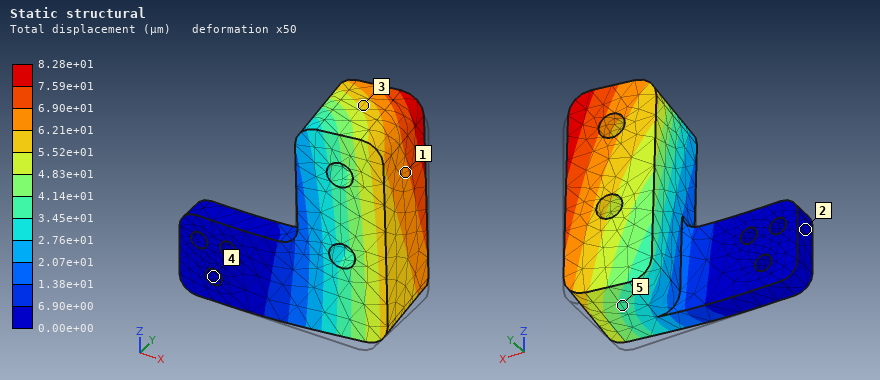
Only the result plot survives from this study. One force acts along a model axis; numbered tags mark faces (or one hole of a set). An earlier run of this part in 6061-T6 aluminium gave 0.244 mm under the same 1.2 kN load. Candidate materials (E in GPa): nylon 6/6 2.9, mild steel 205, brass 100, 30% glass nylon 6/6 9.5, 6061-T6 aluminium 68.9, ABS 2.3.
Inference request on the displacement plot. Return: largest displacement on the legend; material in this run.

8.28e+01 µm
mild steel
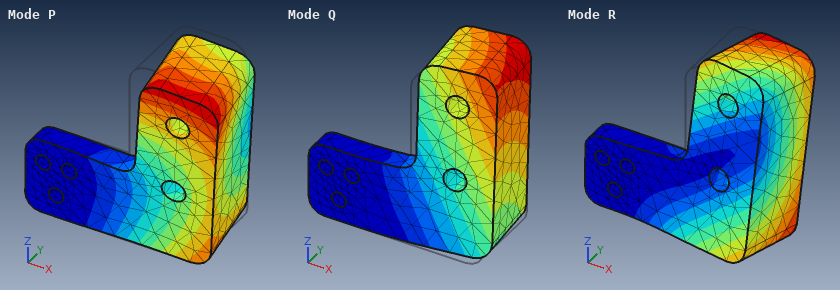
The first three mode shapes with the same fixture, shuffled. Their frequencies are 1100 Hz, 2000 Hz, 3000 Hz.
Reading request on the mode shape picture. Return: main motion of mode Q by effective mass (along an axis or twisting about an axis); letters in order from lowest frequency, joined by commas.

along Y
Q, R, P
